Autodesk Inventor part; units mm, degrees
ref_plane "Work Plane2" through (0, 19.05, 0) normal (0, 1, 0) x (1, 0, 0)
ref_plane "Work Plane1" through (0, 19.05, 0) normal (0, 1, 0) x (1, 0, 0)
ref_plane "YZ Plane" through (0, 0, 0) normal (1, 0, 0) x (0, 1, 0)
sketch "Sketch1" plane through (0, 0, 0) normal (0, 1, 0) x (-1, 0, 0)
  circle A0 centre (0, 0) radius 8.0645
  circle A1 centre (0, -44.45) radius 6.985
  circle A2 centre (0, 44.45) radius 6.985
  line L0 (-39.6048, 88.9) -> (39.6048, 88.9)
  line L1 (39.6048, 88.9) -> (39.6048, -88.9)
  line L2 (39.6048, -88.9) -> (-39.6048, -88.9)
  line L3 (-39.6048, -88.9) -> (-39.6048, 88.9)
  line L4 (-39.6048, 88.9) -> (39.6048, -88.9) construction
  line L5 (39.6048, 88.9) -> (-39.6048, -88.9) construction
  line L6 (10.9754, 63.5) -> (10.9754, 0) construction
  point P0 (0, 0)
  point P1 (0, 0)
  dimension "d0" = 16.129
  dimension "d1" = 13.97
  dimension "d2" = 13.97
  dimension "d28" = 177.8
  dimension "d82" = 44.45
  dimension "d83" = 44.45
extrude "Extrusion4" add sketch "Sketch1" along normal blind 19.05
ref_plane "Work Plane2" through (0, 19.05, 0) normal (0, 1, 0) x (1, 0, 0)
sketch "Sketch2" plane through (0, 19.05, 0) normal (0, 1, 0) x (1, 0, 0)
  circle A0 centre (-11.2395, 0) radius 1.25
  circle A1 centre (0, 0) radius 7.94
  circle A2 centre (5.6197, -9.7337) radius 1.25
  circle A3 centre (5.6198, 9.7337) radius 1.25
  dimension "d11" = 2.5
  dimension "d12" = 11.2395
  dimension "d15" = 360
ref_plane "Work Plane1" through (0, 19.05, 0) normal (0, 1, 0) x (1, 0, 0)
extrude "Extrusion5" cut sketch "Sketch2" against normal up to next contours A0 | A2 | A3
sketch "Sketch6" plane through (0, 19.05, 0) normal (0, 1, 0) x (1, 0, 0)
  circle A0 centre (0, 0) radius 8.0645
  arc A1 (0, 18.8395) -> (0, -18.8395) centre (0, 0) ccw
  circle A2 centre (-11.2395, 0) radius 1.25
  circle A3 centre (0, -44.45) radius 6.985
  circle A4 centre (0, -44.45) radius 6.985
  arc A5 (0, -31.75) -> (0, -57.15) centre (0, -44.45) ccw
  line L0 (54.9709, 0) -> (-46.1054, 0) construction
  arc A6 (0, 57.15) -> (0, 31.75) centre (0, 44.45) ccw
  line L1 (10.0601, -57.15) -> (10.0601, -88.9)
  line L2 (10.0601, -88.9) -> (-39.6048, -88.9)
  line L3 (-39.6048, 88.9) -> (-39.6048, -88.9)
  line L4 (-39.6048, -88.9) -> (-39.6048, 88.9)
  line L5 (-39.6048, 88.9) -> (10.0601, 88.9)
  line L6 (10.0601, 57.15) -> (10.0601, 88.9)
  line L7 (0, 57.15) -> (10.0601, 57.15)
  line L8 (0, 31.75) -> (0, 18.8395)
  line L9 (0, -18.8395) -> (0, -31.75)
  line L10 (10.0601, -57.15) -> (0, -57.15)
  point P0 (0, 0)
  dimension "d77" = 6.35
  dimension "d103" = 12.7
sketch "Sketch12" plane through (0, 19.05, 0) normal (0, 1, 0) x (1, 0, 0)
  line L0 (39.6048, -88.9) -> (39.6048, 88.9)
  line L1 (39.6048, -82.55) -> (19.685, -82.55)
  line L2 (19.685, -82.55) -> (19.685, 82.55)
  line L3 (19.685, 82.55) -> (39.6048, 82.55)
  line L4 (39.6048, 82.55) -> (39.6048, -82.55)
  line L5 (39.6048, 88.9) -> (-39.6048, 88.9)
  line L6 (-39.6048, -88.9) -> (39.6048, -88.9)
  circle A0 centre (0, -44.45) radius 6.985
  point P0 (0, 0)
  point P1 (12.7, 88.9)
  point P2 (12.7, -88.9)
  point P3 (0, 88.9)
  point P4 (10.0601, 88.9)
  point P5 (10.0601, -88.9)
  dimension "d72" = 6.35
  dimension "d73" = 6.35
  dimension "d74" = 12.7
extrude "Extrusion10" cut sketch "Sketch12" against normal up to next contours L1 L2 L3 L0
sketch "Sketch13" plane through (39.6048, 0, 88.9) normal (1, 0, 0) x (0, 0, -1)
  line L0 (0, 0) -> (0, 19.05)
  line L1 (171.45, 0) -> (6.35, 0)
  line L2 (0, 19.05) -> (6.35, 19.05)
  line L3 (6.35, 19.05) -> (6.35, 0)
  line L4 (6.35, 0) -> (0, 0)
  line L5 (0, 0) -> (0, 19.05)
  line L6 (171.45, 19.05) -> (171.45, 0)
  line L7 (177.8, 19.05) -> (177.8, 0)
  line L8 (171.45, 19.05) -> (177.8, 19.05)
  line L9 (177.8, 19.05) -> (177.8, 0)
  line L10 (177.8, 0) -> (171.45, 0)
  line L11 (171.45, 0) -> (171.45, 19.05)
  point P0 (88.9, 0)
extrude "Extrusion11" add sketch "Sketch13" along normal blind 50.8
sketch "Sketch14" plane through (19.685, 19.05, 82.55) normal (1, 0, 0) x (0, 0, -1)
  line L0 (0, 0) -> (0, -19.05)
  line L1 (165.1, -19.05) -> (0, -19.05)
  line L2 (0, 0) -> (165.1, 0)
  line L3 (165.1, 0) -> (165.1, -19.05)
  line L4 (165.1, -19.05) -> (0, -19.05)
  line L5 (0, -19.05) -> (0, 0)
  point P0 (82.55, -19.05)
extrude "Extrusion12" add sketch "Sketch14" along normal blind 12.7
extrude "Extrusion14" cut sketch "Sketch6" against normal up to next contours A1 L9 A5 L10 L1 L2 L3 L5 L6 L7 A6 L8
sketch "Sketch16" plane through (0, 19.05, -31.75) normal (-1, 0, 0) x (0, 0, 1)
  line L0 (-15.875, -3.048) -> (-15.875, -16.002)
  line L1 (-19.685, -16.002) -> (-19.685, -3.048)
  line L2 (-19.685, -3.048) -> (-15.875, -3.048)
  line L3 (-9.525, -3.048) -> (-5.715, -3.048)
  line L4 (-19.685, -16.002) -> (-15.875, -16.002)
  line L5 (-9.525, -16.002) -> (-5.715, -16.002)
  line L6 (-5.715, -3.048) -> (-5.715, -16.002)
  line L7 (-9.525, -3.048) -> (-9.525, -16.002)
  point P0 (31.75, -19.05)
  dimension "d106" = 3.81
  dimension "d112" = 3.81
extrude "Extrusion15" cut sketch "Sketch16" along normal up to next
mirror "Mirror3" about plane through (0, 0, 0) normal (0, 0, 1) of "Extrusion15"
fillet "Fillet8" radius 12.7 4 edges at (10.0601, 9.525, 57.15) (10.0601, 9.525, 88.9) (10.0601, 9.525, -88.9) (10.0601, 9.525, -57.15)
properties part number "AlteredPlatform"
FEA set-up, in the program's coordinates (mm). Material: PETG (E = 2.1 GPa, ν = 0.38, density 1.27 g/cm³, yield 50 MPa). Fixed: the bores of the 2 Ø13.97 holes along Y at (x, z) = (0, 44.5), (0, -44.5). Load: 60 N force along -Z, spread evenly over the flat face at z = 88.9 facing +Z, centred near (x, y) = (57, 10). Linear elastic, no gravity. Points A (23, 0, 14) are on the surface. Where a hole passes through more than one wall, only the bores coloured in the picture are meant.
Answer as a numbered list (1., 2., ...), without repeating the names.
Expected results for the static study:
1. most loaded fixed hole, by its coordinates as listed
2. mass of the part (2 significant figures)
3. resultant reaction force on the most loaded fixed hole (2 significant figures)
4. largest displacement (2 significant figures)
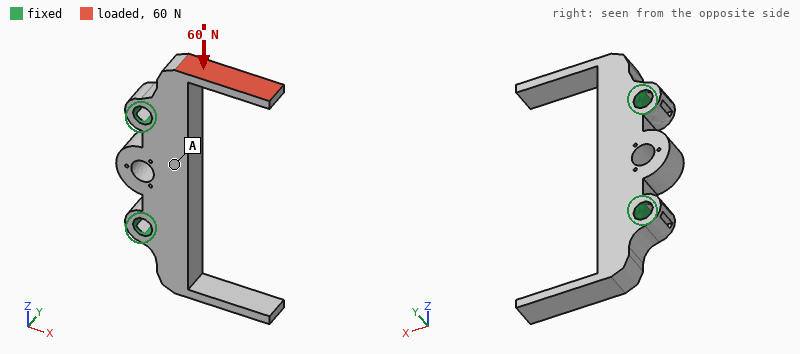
1. (0, -44.5)
2. 150 g
3. 57 N
4. 1.9 mm
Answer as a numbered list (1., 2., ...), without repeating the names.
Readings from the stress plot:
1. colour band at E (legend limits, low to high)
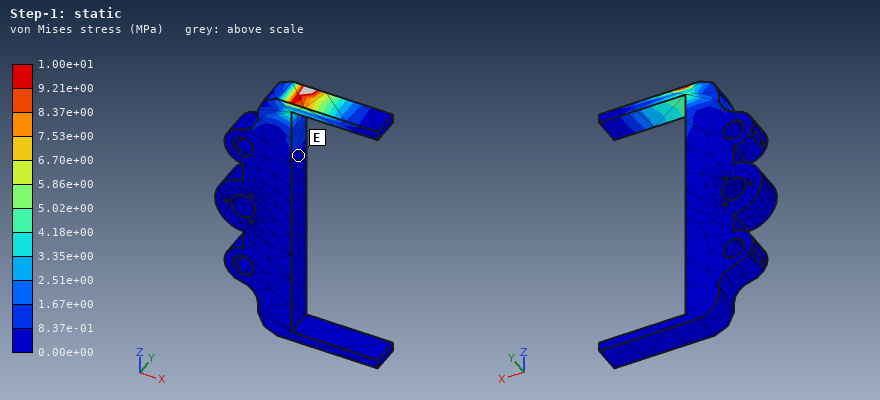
1. 0.00e+00 to 8.37e-01 MPa
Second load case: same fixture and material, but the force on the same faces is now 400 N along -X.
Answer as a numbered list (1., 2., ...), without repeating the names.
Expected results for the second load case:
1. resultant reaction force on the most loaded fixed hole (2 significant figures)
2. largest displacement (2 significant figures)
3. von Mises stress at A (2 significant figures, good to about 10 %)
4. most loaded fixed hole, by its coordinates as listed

1. 580 N
2. 2.4 mm
3. 0.96 MPa
4. (0, 44.5)
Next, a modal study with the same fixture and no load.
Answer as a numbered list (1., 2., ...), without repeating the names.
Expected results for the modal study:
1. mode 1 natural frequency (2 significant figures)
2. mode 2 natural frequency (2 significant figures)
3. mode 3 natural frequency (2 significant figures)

1. 350 Hz
2. 350 Hz
3. 590 Hz
